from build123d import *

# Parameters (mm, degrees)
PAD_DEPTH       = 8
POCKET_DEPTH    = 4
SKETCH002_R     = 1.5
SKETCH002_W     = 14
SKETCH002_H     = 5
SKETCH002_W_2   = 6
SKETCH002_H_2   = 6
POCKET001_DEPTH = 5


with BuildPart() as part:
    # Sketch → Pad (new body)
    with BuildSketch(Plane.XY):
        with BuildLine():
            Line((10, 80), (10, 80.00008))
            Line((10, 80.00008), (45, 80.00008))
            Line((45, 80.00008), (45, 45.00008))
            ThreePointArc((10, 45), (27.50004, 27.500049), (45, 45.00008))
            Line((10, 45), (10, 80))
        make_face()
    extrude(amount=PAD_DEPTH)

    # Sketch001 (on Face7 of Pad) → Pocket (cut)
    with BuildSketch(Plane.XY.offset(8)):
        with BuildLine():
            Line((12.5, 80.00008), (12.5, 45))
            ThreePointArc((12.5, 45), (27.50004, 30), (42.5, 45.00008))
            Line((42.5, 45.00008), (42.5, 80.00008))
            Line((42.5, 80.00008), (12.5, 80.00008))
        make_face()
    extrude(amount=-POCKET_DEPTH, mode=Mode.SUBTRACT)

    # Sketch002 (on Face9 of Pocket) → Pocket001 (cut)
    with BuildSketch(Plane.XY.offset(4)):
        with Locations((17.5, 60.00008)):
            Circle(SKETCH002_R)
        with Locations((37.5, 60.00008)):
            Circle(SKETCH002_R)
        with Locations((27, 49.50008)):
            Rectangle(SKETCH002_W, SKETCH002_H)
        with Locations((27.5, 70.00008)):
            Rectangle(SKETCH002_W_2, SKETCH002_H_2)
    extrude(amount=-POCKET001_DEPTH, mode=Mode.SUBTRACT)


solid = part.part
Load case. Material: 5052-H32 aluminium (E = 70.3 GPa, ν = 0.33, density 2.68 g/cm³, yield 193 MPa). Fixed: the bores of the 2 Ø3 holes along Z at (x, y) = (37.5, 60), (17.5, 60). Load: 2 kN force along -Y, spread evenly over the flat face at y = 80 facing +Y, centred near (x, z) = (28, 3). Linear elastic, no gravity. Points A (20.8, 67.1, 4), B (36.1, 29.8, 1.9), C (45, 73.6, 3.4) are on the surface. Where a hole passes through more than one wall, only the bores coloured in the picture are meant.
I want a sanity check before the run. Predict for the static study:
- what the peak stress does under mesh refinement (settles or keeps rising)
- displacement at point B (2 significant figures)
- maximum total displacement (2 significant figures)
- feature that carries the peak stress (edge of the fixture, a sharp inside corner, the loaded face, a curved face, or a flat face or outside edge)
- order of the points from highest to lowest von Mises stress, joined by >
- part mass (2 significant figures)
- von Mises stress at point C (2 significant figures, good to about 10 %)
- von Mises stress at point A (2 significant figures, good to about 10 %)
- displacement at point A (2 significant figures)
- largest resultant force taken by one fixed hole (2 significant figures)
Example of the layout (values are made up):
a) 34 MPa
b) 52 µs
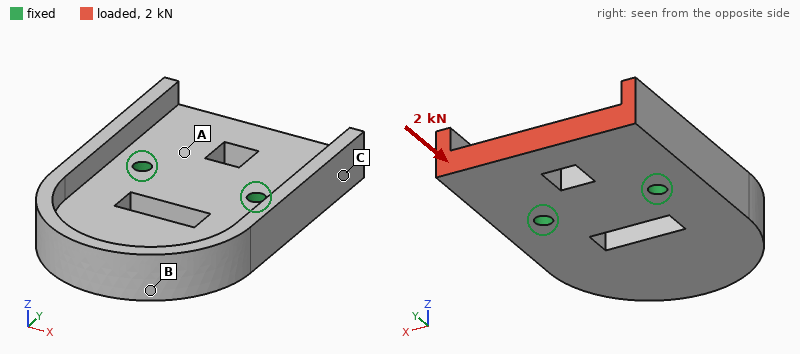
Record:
a) keeps rising
b) 9.6 µm
c) 11 µm
d) edge of the fixture
e) A > C > B
f) 20 g
g) 11 MPa
h) 20 MPa
i) 2.9 µm
j) 1.0 kN
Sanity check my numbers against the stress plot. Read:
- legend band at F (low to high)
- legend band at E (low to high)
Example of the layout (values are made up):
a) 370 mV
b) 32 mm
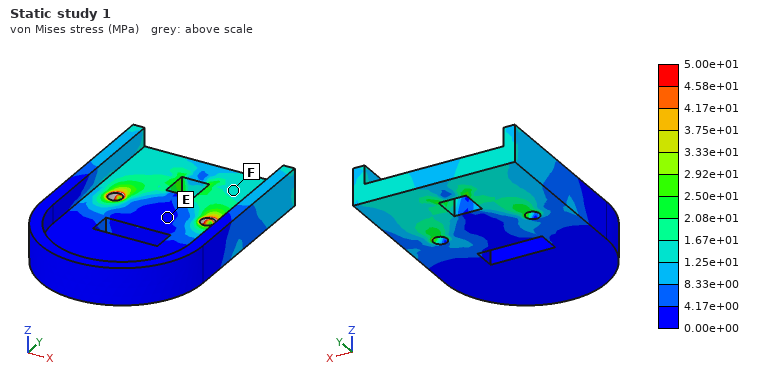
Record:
a) 1.25e+01 to 1.67e+01 MPa
b) 0.00e+00 to 4.17e+00 MPa
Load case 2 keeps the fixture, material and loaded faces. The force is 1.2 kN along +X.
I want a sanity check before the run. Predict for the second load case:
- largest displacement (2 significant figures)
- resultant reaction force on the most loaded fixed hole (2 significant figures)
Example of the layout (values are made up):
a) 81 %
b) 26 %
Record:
a) 33 µm
b) 1.2 kN
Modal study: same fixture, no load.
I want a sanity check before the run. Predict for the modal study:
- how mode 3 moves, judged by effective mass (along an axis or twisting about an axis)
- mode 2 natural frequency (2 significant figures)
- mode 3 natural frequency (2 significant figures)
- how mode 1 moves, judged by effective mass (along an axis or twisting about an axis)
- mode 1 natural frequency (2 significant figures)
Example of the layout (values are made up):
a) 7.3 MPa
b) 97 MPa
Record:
a) along Z
b) 8100 Hz
c) 9000 Hz
d) along Z
e) 3600 Hz
